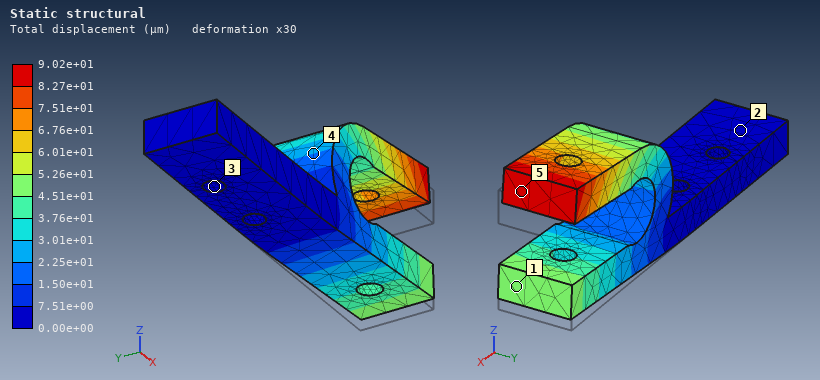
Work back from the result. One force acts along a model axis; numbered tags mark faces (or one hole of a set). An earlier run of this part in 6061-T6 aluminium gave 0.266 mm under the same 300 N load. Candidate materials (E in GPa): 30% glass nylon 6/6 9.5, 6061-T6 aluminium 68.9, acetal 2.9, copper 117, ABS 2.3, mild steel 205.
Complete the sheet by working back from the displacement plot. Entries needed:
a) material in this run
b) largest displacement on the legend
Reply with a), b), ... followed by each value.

a) mild steel
b) 9.02e+01 µm
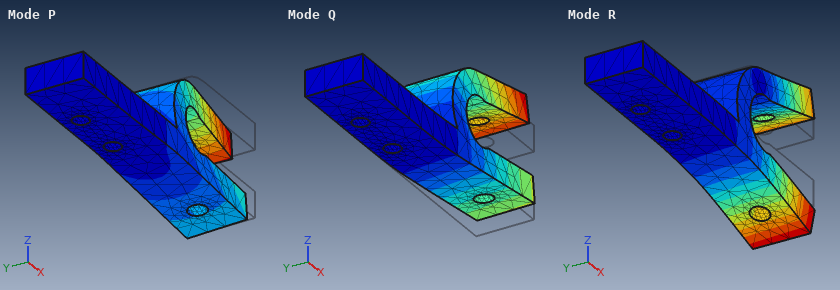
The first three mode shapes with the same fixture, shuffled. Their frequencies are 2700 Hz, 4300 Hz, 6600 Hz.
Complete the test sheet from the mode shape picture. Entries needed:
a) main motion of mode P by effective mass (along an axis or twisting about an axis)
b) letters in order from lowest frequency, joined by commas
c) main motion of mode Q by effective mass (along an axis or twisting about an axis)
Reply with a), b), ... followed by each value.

a) along Y
b) Q, P, R
c) along Z
